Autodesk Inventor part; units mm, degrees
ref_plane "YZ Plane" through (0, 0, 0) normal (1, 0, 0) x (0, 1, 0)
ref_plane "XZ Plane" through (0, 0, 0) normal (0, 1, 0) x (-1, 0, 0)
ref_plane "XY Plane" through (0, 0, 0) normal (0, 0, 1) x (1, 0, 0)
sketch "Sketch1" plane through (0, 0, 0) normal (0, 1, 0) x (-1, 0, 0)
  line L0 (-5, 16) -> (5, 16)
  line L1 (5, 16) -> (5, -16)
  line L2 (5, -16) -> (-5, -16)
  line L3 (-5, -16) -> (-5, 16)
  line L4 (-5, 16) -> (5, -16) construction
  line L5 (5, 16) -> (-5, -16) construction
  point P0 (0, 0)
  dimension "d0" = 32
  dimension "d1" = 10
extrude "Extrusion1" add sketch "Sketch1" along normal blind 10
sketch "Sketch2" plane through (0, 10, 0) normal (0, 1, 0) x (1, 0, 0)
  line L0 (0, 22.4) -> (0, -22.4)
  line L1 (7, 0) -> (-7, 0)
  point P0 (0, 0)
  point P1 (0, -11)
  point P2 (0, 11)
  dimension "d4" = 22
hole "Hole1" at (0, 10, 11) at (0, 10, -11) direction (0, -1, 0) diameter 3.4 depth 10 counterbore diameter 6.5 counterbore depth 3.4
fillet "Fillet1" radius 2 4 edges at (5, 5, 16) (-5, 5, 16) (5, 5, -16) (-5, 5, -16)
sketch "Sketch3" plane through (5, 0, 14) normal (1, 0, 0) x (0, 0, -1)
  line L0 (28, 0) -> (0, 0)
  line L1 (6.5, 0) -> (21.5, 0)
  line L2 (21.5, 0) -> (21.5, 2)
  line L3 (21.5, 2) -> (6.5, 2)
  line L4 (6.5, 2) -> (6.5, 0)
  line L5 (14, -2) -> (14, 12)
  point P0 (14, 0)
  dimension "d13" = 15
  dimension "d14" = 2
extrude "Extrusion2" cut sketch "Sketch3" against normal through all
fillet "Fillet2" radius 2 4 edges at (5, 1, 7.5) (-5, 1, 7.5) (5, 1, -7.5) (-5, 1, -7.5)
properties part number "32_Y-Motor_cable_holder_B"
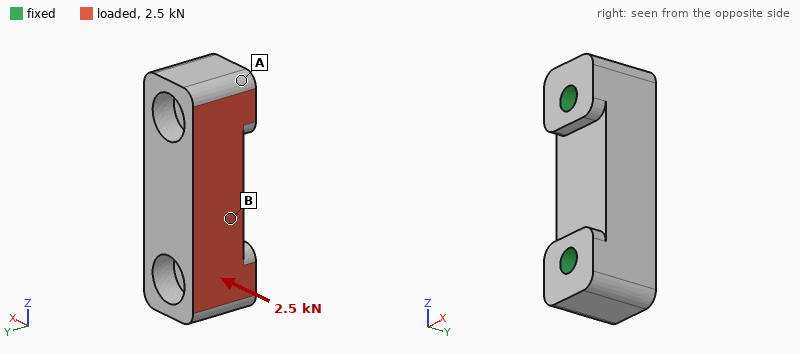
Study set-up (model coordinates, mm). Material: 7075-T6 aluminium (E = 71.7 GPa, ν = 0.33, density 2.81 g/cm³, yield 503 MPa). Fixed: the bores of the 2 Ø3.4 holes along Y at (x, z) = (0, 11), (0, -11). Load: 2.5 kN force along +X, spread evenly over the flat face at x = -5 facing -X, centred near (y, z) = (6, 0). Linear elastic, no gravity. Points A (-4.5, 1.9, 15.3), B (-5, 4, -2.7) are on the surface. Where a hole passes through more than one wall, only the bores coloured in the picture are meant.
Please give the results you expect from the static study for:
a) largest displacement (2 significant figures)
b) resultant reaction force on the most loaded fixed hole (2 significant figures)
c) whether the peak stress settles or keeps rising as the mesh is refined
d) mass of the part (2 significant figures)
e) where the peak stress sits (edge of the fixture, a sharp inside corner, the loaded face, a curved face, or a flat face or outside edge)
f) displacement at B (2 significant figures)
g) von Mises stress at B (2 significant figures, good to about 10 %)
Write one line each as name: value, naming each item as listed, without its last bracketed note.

largest displacement: 8.9 µm
resultant reaction force on the most loaded fixed hole: 1.3 kN
whether the peak stress settles or keeps rising as the mesh is refined: keeps rising
mass of the part: 7.1 g
where the peak stress sits: edge of the fixture
displacement at B: 5.4 µm
von Mises stress at B: 20 MPa
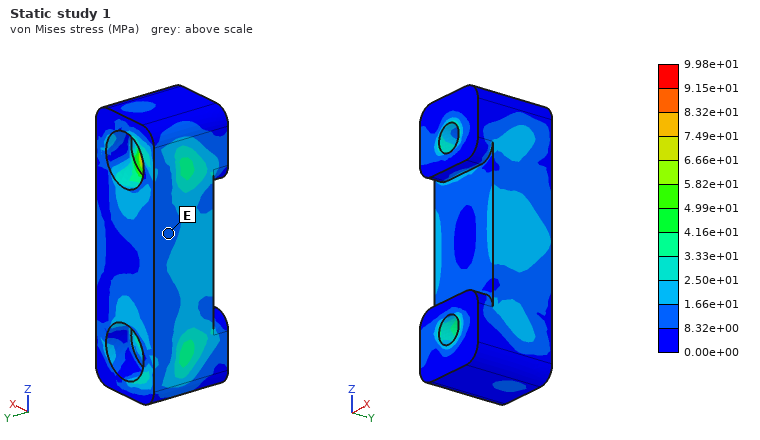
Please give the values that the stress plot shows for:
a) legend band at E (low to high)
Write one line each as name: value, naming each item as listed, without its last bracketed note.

legend band at E: 8.32e+00 to 1.66e+01 MPa
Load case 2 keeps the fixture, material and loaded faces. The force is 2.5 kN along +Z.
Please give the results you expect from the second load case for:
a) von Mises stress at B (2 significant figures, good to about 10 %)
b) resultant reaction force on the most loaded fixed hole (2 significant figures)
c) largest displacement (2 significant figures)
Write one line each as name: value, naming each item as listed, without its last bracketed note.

von Mises stress at B: 21 MPa
resultant reaction force on the most loaded fixed hole: 1.3 kN
largest displacement: 4.4 µm
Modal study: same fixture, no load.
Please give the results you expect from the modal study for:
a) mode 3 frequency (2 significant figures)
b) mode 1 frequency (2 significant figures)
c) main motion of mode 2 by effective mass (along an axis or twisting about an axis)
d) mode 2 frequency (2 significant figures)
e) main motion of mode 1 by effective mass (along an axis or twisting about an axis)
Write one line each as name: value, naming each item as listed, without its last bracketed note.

mode 3 frequency: 59 kHz
mode 1 frequency: 41 kHz
main motion of mode 2 by effective mass: along Y
mode 2 frequency: 50 kHz
main motion of mode 1 by effective mass: along X
